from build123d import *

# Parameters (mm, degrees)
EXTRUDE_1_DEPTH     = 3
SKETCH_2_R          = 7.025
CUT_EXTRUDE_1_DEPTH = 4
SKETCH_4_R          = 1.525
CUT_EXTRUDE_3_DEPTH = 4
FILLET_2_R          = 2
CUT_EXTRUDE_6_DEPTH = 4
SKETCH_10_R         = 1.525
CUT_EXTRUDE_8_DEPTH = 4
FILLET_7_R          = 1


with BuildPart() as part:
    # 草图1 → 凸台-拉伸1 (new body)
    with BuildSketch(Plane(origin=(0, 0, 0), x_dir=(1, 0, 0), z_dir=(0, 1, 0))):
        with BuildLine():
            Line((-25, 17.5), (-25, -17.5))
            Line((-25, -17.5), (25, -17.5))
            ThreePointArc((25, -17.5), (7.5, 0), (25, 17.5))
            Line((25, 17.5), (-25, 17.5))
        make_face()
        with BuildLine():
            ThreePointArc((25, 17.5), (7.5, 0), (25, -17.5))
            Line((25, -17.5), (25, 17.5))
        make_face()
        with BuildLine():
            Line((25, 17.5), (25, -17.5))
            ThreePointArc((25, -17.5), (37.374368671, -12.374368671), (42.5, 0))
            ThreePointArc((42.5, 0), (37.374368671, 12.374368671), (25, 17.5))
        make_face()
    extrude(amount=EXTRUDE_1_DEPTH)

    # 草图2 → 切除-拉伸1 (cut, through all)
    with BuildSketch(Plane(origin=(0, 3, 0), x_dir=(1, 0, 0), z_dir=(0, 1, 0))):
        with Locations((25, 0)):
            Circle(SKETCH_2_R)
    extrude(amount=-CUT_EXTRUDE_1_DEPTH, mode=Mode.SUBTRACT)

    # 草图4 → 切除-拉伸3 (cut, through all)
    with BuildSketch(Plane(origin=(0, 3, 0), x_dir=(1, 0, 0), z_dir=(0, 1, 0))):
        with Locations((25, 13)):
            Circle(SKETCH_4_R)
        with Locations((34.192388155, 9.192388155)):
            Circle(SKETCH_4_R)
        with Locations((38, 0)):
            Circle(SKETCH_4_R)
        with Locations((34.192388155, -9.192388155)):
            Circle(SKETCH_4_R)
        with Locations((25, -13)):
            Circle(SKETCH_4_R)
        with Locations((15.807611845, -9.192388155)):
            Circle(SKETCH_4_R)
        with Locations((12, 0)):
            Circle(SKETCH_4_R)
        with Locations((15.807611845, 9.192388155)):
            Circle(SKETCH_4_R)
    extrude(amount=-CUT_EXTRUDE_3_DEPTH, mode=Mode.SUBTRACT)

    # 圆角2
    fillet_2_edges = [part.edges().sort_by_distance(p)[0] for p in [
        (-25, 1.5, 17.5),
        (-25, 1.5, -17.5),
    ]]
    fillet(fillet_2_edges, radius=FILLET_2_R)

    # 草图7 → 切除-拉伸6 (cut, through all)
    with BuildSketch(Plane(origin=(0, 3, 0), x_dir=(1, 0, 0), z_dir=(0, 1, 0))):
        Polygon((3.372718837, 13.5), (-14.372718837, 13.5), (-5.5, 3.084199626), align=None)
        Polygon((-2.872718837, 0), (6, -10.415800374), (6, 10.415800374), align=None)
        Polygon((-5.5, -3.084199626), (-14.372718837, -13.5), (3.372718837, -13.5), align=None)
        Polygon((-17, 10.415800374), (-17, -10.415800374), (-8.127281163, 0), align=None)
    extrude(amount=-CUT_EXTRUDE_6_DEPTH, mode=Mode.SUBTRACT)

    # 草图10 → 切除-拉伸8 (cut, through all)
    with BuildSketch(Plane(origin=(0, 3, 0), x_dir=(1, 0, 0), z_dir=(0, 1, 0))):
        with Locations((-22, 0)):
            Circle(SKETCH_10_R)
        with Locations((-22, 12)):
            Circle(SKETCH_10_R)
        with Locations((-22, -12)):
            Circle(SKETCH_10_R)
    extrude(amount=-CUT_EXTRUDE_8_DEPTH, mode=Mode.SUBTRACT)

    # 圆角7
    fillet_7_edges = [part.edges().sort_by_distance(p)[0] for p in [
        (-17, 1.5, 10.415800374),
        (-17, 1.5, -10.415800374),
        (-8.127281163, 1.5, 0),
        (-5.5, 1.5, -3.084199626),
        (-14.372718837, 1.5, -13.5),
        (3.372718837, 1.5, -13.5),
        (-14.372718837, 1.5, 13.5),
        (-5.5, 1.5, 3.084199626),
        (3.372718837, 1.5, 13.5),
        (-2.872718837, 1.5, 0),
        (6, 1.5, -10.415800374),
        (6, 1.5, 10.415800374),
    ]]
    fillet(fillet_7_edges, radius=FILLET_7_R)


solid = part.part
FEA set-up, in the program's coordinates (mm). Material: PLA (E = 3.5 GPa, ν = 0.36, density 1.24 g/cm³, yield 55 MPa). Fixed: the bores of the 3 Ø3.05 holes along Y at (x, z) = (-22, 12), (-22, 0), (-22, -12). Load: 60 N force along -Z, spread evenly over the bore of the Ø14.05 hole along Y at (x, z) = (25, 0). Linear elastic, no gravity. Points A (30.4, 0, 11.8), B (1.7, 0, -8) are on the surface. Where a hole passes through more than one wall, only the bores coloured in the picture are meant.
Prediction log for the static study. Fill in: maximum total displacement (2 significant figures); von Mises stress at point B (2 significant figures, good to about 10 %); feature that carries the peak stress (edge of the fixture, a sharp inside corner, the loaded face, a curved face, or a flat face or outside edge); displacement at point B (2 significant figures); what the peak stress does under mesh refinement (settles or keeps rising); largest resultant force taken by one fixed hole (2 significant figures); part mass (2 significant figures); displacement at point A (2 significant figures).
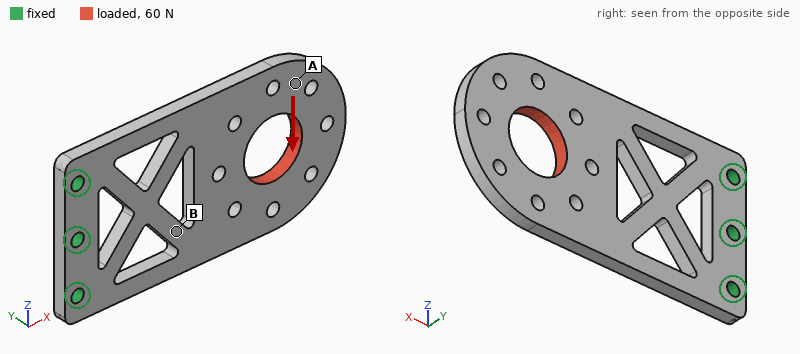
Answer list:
0.23 mm
2.9 MPa
edge of the fixture
0.075 mm
keeps rising
100 N
6.1 g
0.19 mm
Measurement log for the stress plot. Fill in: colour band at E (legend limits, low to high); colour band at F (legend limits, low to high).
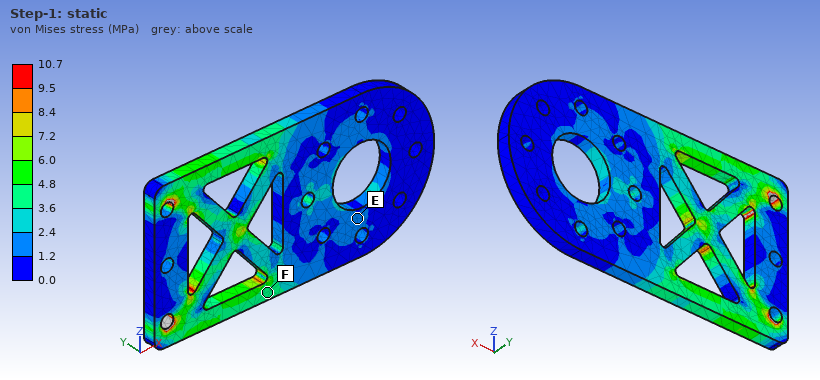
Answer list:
1.2 to 2.4 MPa
3.6 to 4.8 MPa
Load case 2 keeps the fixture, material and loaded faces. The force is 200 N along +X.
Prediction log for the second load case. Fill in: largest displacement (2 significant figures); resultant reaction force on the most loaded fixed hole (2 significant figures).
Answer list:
86 µm
110 N
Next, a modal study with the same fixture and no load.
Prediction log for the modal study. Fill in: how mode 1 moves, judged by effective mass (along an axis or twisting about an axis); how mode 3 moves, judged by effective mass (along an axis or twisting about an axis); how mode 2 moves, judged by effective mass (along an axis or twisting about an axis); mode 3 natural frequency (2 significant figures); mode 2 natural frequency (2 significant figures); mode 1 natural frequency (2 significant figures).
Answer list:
along Y
along Y
twisting about X
1100 Hz
700 Hz
170 Hz
